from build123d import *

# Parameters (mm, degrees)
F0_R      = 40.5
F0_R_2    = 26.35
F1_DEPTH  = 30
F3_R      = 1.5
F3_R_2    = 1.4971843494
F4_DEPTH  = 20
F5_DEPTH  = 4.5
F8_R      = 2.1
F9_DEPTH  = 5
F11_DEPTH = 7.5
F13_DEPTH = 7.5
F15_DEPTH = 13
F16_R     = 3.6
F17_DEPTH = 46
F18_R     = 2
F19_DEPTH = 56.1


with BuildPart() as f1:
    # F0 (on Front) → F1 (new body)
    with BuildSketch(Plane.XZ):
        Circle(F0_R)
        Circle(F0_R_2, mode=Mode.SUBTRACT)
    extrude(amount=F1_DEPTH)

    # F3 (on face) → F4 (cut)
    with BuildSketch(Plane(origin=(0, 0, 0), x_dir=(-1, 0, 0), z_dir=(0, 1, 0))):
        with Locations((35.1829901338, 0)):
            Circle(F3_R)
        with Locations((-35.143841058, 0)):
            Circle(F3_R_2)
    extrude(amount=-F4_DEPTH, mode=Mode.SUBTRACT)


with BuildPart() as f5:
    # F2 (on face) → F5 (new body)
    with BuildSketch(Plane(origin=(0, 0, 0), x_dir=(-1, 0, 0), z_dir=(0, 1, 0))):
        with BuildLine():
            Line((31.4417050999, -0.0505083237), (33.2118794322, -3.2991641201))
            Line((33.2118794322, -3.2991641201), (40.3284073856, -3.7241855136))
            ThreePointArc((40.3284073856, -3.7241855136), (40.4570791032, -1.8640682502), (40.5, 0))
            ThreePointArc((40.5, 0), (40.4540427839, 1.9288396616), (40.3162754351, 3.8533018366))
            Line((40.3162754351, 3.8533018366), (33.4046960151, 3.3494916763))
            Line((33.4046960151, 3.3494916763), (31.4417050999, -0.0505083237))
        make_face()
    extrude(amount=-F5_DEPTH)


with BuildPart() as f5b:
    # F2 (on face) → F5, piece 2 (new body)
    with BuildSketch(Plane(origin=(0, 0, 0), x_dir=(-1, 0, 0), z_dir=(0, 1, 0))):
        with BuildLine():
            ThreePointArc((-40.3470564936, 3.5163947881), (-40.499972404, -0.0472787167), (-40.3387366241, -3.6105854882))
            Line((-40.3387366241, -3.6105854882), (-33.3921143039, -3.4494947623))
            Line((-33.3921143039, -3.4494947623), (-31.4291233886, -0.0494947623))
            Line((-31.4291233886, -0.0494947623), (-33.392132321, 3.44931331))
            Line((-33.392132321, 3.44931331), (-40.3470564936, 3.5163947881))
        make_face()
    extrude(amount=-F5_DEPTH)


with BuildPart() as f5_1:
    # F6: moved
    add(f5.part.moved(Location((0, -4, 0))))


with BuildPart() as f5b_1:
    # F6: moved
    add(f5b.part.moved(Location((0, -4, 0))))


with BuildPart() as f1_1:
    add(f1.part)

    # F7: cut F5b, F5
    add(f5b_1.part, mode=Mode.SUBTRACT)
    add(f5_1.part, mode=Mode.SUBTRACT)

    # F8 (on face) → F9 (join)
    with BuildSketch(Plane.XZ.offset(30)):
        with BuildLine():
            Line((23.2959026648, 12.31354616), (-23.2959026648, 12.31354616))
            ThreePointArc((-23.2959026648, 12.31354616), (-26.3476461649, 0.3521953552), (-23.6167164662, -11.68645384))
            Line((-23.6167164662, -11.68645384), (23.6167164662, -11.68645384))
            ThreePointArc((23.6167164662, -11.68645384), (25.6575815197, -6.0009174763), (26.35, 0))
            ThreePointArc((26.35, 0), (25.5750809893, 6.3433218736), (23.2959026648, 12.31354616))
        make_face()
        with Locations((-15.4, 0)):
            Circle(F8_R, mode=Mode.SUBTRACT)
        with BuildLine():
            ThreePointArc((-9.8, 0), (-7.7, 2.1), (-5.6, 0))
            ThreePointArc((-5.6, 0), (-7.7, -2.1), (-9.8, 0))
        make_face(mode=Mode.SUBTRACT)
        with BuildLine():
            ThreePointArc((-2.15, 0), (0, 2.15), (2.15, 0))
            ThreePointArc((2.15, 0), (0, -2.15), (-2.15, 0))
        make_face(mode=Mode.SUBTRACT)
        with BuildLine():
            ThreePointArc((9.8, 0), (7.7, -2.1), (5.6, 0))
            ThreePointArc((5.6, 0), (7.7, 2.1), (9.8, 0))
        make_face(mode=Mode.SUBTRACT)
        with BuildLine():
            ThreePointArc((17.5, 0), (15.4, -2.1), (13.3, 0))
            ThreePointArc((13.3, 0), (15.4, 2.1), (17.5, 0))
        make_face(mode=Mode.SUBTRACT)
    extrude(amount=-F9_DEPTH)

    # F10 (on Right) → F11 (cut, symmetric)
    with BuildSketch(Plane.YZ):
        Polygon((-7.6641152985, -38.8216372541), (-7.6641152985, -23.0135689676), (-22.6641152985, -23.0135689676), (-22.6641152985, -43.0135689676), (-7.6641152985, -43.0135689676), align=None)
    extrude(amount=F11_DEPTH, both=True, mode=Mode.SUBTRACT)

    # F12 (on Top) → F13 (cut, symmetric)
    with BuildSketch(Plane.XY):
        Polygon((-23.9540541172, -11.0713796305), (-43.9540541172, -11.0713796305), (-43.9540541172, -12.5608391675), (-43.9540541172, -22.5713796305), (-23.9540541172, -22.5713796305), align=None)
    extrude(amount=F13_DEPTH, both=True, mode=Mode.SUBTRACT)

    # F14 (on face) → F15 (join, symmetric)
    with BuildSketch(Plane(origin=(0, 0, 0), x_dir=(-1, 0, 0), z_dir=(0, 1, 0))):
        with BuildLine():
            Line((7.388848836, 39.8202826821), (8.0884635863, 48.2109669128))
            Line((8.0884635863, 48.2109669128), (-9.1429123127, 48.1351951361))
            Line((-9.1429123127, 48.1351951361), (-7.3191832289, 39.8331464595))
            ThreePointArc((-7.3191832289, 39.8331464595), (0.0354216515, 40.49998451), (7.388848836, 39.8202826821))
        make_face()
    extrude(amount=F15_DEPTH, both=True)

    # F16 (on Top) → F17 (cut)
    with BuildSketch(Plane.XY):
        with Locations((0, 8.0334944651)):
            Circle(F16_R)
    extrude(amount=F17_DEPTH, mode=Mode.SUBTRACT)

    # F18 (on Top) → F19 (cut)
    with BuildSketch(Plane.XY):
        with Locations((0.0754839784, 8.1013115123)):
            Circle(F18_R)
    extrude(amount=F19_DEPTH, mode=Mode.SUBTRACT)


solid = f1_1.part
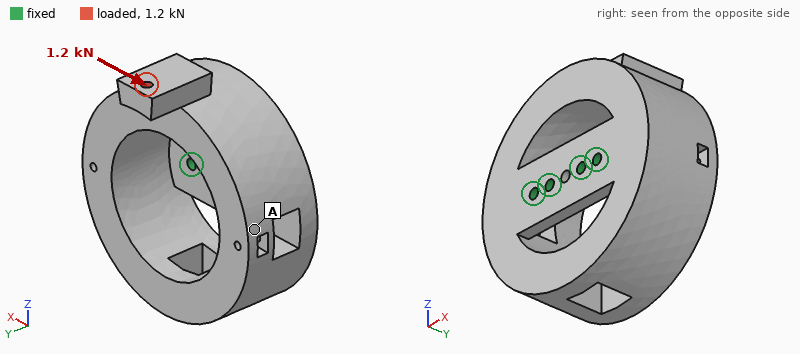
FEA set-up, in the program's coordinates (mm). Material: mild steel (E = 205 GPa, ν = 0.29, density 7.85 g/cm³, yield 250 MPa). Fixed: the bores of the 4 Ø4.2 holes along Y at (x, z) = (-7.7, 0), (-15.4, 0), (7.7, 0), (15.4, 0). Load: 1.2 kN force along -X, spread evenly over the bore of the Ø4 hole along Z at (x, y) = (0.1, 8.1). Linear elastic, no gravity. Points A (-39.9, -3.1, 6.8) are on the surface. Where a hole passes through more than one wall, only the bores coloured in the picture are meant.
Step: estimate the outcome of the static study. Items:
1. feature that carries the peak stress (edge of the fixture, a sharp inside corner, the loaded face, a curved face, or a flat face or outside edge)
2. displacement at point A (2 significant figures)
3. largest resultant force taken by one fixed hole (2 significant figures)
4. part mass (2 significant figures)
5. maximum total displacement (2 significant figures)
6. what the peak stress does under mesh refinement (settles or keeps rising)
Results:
edge of the fixture
18 µm
2.0 kN
720 g
33 µm
keeps rising
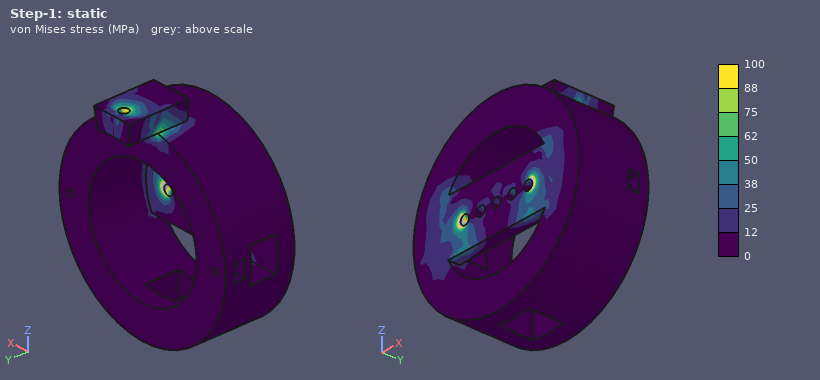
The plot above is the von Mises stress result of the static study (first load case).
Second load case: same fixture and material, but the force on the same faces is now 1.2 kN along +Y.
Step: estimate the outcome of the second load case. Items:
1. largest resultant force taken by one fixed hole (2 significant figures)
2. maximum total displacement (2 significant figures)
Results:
650 N
0.22 mm
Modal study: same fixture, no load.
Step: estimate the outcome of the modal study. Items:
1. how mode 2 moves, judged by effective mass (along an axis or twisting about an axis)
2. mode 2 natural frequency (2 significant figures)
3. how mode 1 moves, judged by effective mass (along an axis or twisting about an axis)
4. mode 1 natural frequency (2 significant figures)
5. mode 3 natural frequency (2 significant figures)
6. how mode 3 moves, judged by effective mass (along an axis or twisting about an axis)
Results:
along X
2500 Hz
along Z
860 Hz
3100 Hz
twisting about Y
